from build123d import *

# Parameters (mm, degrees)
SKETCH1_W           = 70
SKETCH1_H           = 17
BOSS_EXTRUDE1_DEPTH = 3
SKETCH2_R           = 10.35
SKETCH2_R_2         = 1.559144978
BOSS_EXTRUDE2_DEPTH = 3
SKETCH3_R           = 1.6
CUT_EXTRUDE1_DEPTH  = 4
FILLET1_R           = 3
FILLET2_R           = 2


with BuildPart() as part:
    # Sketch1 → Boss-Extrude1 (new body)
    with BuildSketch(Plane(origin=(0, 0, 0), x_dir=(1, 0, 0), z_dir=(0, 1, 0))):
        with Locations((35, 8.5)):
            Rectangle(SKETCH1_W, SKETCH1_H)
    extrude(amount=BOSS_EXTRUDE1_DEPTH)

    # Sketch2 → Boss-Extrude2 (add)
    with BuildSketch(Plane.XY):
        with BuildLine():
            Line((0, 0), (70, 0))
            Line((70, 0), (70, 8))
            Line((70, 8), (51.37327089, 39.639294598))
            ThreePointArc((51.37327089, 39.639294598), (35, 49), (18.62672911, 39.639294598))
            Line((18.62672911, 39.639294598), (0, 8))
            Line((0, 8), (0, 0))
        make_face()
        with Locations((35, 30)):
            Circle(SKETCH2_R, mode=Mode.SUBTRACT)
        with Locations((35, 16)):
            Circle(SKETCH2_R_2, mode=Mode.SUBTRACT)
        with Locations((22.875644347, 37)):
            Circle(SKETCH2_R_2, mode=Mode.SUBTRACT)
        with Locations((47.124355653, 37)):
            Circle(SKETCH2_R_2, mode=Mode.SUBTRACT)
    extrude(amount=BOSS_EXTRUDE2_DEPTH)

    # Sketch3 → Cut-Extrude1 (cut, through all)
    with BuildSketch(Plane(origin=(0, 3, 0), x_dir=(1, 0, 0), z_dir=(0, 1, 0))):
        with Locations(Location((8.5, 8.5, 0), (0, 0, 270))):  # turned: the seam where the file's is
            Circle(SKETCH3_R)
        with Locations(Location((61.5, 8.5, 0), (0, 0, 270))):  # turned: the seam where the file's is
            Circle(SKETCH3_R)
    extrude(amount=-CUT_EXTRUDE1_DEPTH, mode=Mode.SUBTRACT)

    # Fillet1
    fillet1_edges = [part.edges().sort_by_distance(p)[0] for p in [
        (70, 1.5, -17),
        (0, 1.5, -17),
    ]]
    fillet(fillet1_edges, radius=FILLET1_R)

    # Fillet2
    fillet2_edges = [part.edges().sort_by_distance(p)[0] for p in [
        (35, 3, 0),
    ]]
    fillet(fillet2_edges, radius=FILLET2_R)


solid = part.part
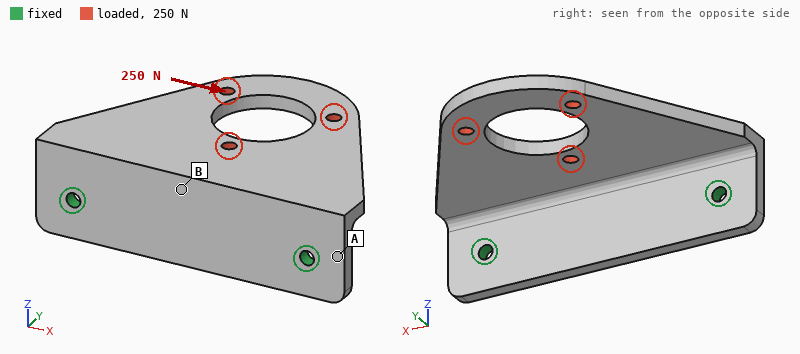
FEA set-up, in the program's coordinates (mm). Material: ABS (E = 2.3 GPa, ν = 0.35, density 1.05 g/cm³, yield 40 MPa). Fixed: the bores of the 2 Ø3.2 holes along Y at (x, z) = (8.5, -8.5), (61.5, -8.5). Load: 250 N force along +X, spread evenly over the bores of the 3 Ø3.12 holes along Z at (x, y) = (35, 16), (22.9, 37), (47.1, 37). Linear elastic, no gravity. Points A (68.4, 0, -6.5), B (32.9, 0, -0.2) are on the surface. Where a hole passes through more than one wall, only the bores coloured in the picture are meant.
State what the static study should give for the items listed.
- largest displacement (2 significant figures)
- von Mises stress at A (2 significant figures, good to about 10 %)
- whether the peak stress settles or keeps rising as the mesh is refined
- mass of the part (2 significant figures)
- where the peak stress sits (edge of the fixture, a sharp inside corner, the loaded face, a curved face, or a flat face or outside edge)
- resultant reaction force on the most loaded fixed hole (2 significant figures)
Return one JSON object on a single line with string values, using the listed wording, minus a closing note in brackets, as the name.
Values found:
{"largest displacement": "0.87 mm", "von Mises stress at A": "16 MPa", "whether the peak stress settles or keeps rising as the mesh is refined": "keeps rising", "mass of the part": "10 g", "where the peak stress sits": "edge of the fixture", "resultant reaction force on the most loaded fixed hole": "190 N"}
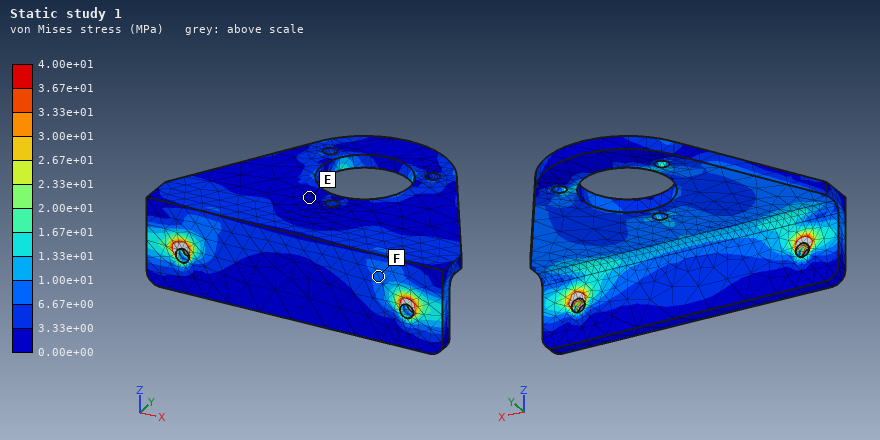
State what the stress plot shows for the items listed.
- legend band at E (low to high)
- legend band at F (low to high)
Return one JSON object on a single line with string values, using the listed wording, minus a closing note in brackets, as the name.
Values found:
{"legend band at E": "0.00e+00 to 3.33e+00 MPa", "legend band at F": "6.67e+00 to 1.00e+01 MPa"}
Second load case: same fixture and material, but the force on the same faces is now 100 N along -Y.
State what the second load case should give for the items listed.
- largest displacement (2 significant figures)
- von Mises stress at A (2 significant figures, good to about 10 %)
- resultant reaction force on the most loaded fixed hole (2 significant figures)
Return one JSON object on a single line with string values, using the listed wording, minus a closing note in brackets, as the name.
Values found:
{"largest displacement": "1.0 mm", "von Mises stress at A": "7.2 MPa", "resultant reaction force on the most loaded fixed hole": "51 N"}
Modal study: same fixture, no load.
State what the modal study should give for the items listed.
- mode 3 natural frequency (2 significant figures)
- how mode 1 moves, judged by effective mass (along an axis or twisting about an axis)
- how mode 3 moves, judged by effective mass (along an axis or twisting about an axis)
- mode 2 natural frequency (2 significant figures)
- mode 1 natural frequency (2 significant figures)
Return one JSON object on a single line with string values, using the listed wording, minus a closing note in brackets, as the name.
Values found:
{"mode 3 natural frequency": "1300 Hz", "how mode 1 moves, judged by effective mass": "along Z", "how mode 3 moves, judged by effective mass": "along Y", "mode 2 natural frequency": "980 Hz", "mode 1 natural frequency": "360 Hz"}
